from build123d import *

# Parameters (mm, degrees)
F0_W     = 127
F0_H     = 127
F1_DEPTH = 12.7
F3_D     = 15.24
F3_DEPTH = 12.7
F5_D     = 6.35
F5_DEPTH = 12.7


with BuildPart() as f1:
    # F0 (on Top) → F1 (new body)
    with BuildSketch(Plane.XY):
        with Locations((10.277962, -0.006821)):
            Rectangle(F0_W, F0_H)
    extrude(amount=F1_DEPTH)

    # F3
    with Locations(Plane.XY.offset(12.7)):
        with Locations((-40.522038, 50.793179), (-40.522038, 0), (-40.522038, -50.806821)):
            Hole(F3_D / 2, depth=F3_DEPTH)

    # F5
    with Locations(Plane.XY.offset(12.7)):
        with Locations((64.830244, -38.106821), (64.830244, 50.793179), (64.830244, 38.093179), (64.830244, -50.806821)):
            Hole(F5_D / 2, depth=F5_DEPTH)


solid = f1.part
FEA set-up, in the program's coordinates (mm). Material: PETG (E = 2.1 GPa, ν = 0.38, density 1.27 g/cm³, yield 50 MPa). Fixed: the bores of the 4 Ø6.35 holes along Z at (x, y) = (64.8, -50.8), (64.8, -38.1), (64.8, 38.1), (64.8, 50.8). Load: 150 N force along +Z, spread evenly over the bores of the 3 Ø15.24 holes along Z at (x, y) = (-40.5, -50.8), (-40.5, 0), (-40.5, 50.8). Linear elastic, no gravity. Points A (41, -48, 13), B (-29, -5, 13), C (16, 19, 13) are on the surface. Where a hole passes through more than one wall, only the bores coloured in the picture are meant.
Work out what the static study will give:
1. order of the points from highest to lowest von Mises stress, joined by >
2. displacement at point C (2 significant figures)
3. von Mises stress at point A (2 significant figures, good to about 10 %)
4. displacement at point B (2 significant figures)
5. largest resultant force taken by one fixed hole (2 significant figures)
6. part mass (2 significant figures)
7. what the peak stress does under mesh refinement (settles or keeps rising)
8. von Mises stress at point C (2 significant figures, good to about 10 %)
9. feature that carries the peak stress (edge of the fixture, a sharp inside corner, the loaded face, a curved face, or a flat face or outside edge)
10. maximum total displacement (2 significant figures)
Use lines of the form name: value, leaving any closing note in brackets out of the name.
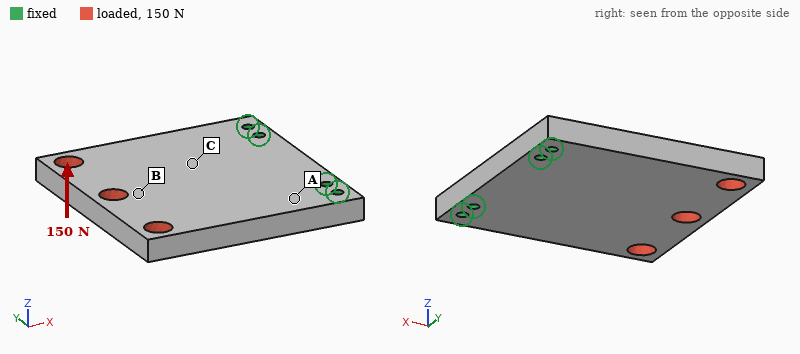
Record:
order of the points from highest to lowest von Mises stress, joined by >: A > C > B
displacement at point C: 0.48 mm
von Mises stress at point A: 4.0 MPa
displacement at point B: 1.3 mm
largest resultant force taken by one fixed hole: 73 N
part mass: 250 g
what the peak stress does under mesh refinement: keeps rising
von Mises stress at point C: 2.2 MPa
feature that carries the peak stress: edge of the fixture
maximum total displacement: 1.8 mm
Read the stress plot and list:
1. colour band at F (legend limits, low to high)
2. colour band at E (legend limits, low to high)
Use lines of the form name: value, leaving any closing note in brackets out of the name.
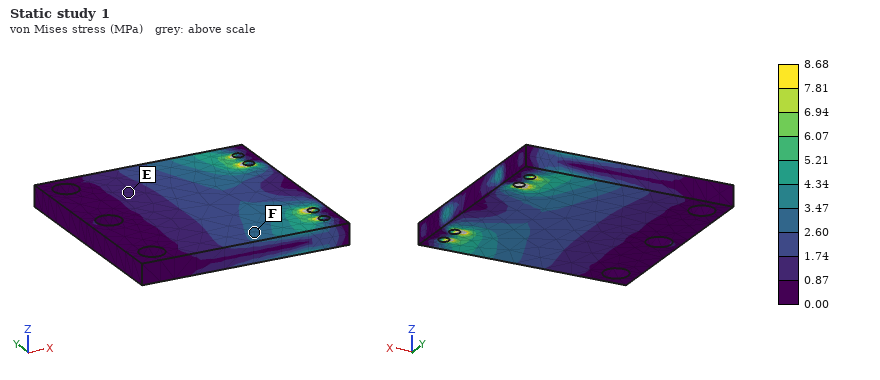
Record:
colour band at F: 2.60 to 3.47 MPa
colour band at E: 0.87 to 1.74 MPa
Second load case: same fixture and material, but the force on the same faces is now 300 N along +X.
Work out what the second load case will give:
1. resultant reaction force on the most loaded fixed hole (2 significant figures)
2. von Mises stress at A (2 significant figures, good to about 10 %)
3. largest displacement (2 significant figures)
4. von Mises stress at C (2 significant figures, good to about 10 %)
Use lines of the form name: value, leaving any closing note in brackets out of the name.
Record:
resultant reaction force on the most loaded fixed hole: 85 N
von Mises stress at A: 0.28 MPa
largest displacement: 18 µm
von Mises stress at C: 0.14 MPa
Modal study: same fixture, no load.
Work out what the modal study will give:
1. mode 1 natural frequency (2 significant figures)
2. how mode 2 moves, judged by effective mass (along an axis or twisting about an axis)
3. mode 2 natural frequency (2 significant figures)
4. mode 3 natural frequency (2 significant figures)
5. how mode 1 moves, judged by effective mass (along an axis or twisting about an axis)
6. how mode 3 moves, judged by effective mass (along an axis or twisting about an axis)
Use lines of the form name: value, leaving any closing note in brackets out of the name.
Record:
mode 1 natural frequency: 180 Hz
how mode 2 moves, judged by effective mass: twisting about X
mode 2 natural frequency: 440 Hz
mode 3 natural frequency: 1100 Hz
how mode 1 moves, judged by effective mass: along Z
how mode 3 moves, judged by effective mass: along Z
